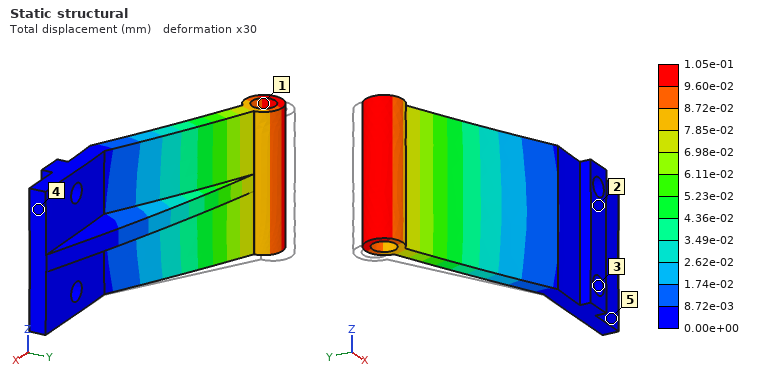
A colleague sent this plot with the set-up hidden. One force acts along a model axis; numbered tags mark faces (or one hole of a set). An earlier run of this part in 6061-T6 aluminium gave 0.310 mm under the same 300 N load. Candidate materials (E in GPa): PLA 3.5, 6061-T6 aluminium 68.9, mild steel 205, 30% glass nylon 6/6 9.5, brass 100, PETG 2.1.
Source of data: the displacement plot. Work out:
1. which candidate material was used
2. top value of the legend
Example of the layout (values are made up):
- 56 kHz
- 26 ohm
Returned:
- mild steel
- 1.05e-01 mm
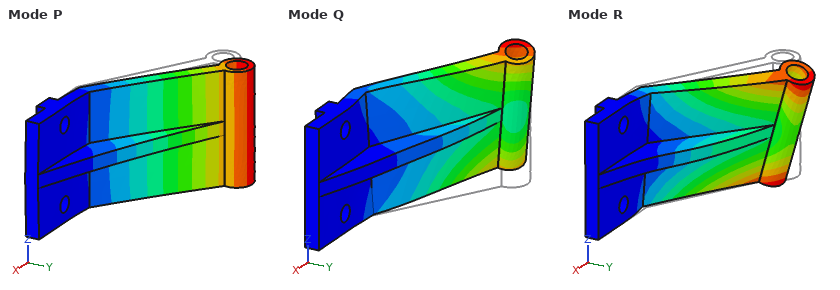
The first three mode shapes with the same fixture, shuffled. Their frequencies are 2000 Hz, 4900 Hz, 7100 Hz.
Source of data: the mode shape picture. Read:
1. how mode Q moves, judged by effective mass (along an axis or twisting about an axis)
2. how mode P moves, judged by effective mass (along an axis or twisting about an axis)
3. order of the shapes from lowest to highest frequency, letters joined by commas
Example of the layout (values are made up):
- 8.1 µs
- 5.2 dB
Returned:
- along Z
- along Y
- P, R, Q
